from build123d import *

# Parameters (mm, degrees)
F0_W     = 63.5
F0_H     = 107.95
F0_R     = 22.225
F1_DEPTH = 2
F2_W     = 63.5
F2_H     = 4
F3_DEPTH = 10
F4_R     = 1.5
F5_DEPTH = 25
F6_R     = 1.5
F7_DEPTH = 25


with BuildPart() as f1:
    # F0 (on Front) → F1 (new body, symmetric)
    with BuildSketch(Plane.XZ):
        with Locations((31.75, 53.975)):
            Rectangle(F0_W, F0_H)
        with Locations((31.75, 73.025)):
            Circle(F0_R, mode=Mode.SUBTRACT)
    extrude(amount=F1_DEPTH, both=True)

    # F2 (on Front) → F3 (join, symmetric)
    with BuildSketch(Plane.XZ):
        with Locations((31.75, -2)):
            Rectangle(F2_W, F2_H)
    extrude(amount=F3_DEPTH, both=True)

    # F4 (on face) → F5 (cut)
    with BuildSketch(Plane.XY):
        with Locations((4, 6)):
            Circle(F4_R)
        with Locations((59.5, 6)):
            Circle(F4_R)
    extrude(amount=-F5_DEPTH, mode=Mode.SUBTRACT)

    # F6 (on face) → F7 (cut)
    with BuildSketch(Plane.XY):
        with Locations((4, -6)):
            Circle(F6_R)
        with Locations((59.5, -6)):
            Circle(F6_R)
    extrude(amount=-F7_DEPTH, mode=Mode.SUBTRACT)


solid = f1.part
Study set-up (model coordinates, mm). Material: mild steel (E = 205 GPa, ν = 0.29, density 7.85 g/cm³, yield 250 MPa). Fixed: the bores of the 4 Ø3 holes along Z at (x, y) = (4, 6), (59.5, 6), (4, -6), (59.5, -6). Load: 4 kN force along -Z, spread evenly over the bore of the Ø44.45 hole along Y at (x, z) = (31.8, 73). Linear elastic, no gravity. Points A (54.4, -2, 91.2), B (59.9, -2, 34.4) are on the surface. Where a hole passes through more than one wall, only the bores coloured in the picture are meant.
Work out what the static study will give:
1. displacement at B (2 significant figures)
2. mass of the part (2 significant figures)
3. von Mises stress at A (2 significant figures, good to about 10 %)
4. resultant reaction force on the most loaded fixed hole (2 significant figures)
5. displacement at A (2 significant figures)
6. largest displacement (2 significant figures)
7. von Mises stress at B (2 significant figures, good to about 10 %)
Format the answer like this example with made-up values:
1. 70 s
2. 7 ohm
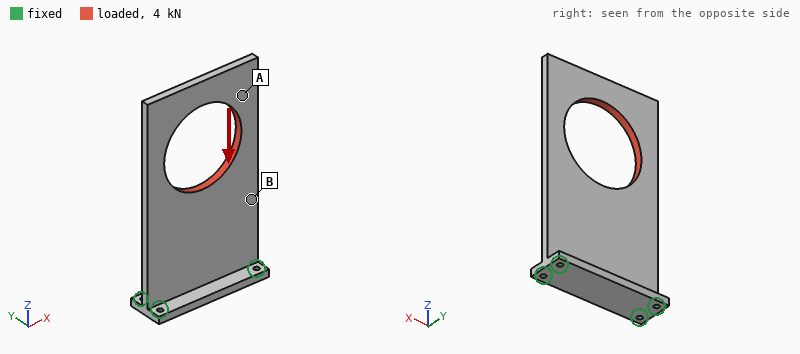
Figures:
1. 7.5 µm
2. 210 g
3. 13 MPa
4. 1.1 kN
5. 16 µm
6. 23 µm
7. 28 MPa
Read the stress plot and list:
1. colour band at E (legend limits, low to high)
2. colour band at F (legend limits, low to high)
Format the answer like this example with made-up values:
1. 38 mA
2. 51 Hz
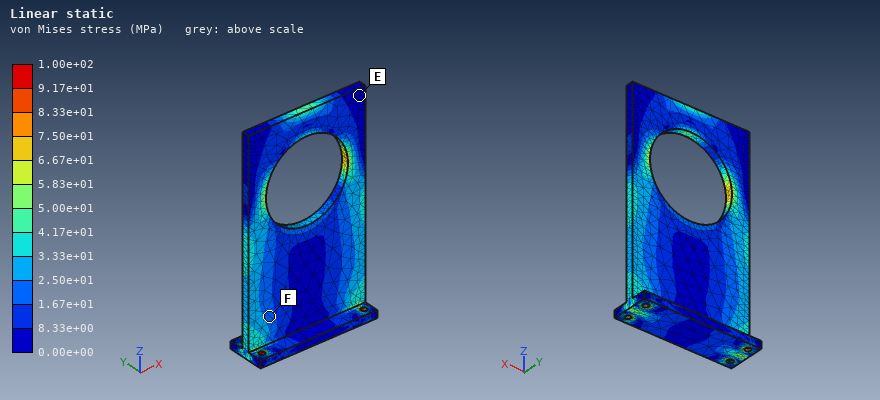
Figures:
1. 0.00e+00 to 8.33e+00 MPa
2. 1.67e+01 to 2.50e+01 MPa
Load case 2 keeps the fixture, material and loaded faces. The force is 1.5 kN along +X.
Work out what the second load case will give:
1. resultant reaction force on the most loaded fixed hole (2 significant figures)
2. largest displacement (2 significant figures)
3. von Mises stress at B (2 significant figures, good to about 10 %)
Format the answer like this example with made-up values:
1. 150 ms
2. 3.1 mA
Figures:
1. 1.1 kN
2. 64 µm
3. 24 MPa
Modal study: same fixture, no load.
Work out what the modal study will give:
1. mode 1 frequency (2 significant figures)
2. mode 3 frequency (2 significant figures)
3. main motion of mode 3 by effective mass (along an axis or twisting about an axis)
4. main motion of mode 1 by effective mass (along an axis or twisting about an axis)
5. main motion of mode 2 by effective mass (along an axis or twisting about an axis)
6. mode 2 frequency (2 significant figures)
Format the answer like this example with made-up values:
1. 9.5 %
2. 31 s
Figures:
1. 300 Hz
2. 1400 Hz
3. along Y
4. along Y
5. twisting about Z
6. 950 Hz
